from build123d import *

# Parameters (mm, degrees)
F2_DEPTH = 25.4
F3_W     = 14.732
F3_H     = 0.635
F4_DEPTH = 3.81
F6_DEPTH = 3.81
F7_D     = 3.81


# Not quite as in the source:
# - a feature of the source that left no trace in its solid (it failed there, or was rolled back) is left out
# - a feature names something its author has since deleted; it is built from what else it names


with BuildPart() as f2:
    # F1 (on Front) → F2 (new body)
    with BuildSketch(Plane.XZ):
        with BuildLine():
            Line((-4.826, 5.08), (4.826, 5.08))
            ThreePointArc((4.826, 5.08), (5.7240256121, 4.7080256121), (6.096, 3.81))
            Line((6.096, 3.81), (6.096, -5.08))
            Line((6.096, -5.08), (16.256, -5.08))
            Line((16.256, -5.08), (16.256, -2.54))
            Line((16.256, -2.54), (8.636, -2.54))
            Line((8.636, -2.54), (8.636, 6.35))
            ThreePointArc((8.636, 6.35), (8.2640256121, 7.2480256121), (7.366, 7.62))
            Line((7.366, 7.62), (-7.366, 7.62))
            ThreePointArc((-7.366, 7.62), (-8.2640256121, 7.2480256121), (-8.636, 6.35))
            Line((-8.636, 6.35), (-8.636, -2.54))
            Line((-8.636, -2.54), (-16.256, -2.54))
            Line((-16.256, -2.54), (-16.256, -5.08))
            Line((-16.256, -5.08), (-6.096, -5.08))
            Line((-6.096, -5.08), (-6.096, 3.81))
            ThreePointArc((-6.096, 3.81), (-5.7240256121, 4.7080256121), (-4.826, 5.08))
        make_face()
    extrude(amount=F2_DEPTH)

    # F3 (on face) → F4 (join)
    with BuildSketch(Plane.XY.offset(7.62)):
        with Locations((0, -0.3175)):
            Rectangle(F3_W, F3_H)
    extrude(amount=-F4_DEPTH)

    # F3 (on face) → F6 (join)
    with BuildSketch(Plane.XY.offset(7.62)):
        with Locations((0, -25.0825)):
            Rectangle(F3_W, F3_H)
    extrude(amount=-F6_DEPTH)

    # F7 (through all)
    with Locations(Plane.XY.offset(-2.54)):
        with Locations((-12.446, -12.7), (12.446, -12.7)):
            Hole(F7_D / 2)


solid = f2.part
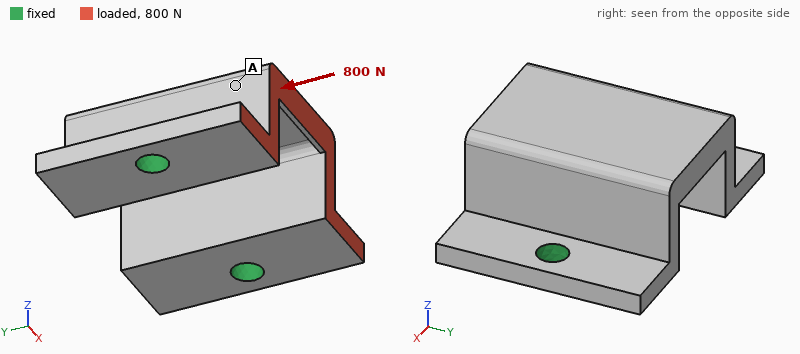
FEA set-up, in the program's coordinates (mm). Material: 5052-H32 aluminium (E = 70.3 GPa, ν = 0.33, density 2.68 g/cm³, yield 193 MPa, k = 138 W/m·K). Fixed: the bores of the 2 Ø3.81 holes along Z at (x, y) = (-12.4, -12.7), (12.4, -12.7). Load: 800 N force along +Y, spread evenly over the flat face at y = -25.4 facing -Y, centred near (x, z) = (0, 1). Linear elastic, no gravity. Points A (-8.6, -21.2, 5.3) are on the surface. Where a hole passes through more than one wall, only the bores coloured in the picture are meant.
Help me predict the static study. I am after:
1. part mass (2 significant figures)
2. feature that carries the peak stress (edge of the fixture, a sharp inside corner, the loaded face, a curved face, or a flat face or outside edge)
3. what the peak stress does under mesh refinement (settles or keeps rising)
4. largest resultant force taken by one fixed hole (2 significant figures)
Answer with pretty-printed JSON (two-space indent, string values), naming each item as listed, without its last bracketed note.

{
  "part mass": "9.0 g",
  "feature that carries the peak stress": "edge of the fixture",
  "what the peak stress does under mesh refinement": "keeps rising",
  "largest resultant force taken by one fixed hole": "400 N"
}
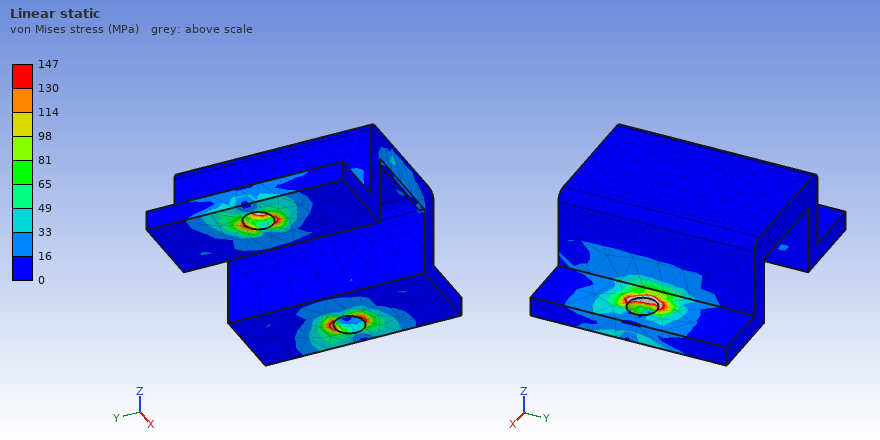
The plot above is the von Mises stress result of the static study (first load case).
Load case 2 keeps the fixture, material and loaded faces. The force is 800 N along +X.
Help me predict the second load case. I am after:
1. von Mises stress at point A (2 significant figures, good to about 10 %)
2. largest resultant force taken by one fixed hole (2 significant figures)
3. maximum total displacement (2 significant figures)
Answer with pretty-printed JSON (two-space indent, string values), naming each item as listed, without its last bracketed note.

{
  "von Mises stress at point A": "45 MPa",
  "largest resultant force taken by one fixed hole": "480 N",
  "maximum total displacement": "46 µm"
}
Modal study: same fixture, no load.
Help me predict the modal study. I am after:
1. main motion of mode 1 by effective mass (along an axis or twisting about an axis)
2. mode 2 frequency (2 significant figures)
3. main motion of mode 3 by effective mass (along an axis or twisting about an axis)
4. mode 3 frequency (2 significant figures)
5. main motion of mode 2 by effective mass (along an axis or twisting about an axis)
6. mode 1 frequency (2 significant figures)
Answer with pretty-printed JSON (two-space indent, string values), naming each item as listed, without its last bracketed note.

{
  "main motion of mode 1 by effective mass": "along Y",
  "mode 2 frequency": "13 kHz",
  "main motion of mode 3 by effective mass": "twisting about Z",
  "mode 3 frequency": "14 kHz",
  "main motion of mode 2 by effective mass": "along X",
  "mode 1 frequency": "6800 Hz"
}
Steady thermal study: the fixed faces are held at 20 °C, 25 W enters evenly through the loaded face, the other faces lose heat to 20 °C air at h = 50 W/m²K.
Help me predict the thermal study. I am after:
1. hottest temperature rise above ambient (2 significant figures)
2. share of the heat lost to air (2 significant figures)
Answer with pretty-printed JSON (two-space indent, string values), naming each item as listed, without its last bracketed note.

{
  "hottest temperature rise above ambient": "33 K",
  "share of the heat lost to air": "7.1 %"
}
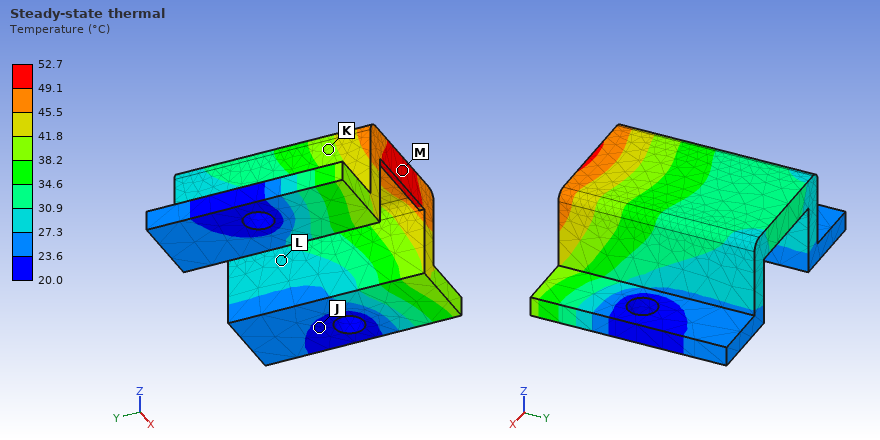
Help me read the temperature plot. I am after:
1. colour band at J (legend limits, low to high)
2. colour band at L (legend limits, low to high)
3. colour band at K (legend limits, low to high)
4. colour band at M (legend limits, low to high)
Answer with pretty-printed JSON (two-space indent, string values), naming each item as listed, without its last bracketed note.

{
  "colour band at J": "20.0 to 23.6 °C",
  "colour band at L": "27.3 to 30.9 °C",
  "colour band at K": "38.2 to 41.8 °C",
  "colour band at M": "49.1 to 52.7 °C"
}
